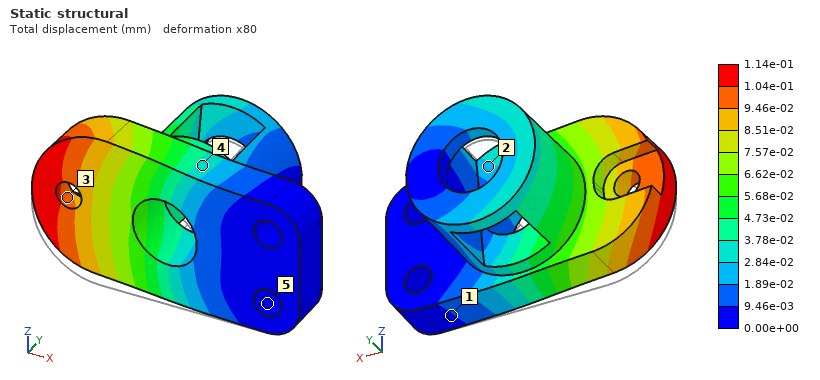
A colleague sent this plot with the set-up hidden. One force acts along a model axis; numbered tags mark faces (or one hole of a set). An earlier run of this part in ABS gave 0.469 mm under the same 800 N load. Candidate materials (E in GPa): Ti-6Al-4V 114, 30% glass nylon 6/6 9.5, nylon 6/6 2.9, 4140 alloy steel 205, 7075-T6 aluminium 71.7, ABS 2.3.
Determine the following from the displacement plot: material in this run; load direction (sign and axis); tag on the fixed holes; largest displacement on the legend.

30% glass nylon 6/6
+Z
5
1.14e-01 mm
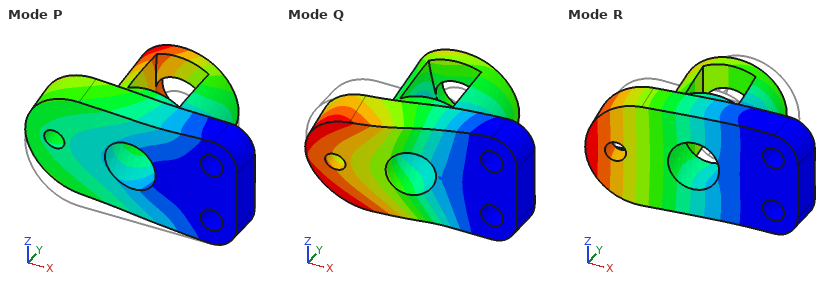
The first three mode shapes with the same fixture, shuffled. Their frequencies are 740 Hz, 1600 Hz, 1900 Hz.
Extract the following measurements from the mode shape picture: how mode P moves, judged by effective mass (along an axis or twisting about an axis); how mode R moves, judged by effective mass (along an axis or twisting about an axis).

along Z
along Y
